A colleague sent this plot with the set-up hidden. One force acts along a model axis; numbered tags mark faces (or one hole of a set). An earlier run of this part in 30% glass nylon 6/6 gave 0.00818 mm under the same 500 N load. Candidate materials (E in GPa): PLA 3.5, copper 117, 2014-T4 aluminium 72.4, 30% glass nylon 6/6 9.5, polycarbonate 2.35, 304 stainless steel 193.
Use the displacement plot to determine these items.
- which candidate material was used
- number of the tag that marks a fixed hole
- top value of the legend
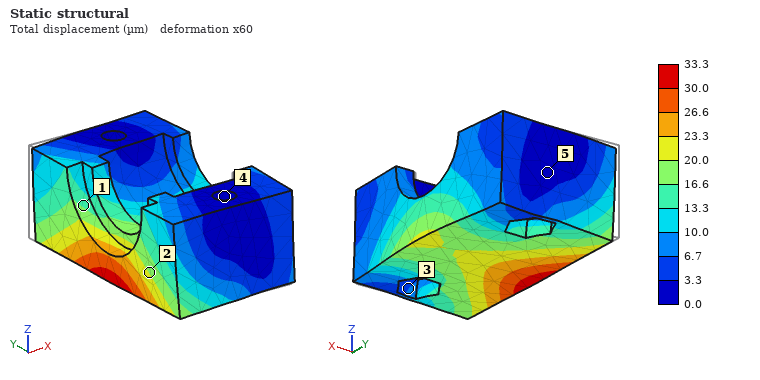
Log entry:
polycarbonate
4
33.3 µm
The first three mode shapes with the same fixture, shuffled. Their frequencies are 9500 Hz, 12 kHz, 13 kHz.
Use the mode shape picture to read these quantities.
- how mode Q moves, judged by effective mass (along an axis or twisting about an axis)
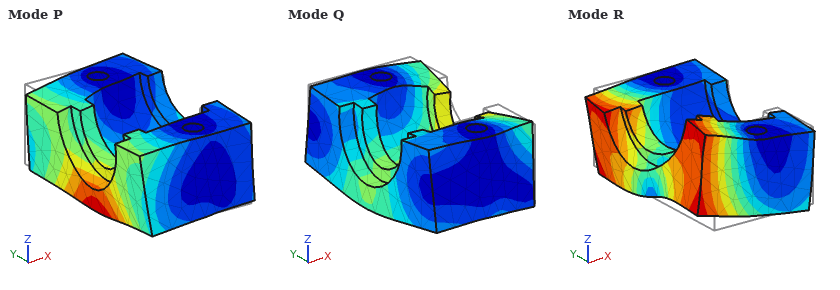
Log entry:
along Z
